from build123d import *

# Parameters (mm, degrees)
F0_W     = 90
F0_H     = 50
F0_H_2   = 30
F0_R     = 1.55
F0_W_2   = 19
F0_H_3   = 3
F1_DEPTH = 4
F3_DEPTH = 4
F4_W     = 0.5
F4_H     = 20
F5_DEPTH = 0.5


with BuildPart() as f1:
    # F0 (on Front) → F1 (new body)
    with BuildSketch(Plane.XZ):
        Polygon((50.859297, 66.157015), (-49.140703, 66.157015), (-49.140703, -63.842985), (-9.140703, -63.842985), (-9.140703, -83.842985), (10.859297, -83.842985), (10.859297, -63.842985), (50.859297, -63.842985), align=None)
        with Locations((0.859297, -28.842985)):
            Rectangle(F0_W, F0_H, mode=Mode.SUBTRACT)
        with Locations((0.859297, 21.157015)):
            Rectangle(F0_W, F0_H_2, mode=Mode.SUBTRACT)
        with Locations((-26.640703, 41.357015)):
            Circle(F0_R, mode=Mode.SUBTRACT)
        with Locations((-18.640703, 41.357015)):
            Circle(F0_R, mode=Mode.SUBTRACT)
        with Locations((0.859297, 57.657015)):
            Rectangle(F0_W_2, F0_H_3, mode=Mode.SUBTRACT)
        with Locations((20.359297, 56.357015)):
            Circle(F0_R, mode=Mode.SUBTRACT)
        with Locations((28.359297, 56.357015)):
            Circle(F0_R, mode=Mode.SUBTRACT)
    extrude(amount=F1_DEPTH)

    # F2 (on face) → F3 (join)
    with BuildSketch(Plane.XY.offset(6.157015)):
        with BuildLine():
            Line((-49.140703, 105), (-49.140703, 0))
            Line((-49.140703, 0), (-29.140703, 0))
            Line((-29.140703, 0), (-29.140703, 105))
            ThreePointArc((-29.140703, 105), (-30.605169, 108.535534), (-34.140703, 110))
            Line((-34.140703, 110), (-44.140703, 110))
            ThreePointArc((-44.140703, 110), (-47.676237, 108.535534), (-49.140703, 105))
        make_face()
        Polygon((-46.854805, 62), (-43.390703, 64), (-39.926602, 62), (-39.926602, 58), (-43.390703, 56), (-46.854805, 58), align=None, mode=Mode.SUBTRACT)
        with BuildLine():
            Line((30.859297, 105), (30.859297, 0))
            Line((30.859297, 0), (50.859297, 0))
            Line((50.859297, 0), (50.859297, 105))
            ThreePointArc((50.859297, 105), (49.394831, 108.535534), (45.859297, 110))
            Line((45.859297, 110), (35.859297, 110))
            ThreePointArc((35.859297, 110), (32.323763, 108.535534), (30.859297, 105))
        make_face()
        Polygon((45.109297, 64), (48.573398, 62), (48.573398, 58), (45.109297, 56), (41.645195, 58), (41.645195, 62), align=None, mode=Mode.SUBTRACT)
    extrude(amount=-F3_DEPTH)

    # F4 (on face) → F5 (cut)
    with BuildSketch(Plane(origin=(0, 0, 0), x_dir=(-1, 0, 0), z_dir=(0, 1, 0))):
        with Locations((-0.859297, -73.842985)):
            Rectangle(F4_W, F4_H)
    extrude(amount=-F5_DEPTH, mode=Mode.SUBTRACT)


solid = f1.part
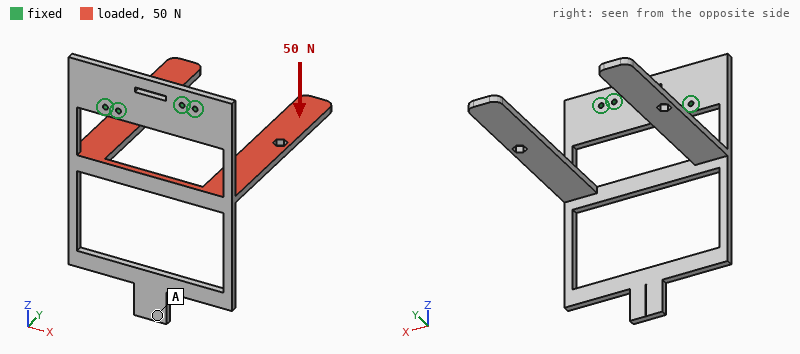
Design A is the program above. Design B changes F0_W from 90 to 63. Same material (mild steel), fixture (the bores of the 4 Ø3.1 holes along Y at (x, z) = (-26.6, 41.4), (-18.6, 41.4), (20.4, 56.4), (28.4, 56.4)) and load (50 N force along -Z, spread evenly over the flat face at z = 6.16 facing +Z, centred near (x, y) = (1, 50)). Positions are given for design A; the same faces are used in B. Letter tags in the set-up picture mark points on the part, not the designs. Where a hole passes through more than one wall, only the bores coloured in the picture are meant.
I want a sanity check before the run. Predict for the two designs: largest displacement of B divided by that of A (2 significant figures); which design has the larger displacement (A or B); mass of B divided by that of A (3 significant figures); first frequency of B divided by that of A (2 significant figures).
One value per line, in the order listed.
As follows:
0.41
A
1.21
1.6
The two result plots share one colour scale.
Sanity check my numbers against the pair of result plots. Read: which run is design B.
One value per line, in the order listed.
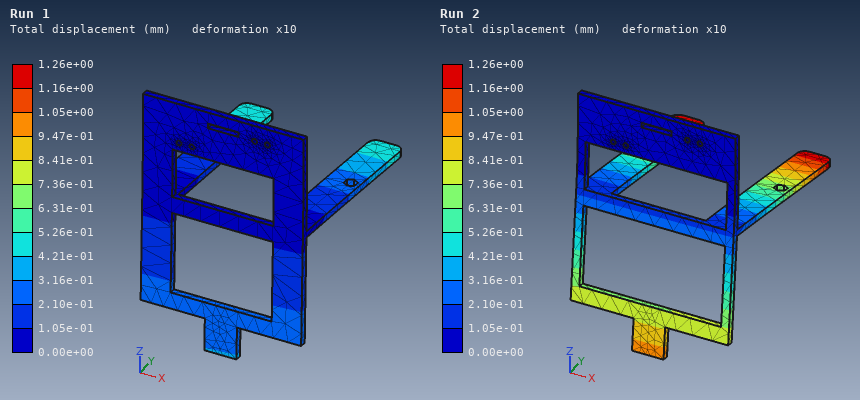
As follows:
Run 1
